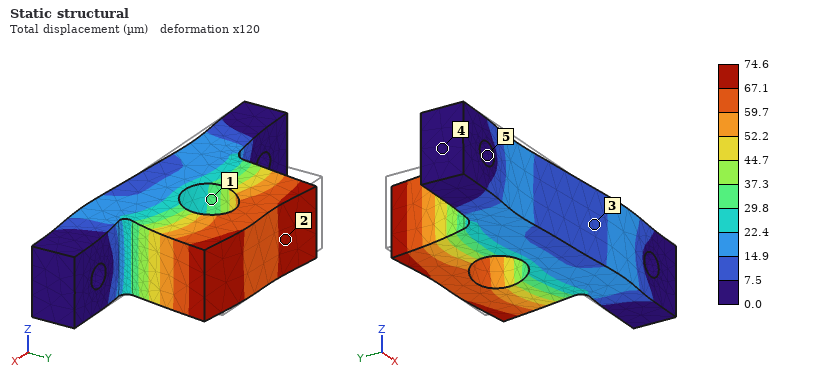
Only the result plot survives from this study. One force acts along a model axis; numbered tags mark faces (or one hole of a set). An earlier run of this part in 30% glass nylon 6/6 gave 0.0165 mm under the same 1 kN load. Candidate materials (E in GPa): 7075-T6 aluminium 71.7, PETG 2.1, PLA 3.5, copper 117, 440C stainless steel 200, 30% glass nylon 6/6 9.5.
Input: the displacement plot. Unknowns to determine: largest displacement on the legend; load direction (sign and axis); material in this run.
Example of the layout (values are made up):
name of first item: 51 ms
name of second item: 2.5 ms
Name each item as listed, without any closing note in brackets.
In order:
largest displacement on the legend: 74.6 µm
load direction: +X
material in this run: PETG
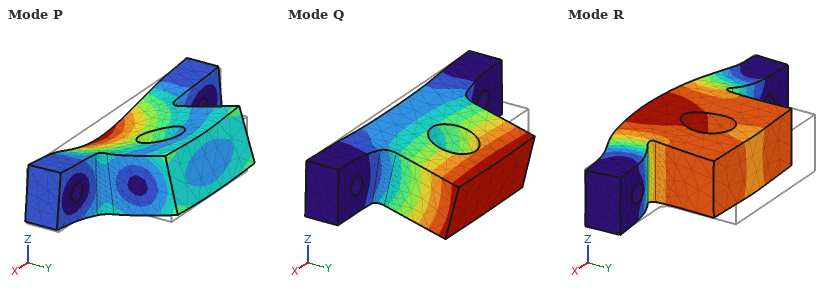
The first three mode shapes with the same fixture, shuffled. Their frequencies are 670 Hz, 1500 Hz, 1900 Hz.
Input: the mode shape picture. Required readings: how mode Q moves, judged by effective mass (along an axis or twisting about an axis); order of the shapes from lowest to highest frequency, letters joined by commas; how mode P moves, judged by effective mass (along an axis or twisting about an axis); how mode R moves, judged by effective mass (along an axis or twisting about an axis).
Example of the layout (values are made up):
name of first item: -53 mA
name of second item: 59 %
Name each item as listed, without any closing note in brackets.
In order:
how mode Q moves, judged by effective mass: along Z
order of the shapes from lowest to highest frequency, letters joined by commas: Q, R, P
how mode P moves, judged by effective mass: along Z
how mode R moves, judged by effective mass: along Y
